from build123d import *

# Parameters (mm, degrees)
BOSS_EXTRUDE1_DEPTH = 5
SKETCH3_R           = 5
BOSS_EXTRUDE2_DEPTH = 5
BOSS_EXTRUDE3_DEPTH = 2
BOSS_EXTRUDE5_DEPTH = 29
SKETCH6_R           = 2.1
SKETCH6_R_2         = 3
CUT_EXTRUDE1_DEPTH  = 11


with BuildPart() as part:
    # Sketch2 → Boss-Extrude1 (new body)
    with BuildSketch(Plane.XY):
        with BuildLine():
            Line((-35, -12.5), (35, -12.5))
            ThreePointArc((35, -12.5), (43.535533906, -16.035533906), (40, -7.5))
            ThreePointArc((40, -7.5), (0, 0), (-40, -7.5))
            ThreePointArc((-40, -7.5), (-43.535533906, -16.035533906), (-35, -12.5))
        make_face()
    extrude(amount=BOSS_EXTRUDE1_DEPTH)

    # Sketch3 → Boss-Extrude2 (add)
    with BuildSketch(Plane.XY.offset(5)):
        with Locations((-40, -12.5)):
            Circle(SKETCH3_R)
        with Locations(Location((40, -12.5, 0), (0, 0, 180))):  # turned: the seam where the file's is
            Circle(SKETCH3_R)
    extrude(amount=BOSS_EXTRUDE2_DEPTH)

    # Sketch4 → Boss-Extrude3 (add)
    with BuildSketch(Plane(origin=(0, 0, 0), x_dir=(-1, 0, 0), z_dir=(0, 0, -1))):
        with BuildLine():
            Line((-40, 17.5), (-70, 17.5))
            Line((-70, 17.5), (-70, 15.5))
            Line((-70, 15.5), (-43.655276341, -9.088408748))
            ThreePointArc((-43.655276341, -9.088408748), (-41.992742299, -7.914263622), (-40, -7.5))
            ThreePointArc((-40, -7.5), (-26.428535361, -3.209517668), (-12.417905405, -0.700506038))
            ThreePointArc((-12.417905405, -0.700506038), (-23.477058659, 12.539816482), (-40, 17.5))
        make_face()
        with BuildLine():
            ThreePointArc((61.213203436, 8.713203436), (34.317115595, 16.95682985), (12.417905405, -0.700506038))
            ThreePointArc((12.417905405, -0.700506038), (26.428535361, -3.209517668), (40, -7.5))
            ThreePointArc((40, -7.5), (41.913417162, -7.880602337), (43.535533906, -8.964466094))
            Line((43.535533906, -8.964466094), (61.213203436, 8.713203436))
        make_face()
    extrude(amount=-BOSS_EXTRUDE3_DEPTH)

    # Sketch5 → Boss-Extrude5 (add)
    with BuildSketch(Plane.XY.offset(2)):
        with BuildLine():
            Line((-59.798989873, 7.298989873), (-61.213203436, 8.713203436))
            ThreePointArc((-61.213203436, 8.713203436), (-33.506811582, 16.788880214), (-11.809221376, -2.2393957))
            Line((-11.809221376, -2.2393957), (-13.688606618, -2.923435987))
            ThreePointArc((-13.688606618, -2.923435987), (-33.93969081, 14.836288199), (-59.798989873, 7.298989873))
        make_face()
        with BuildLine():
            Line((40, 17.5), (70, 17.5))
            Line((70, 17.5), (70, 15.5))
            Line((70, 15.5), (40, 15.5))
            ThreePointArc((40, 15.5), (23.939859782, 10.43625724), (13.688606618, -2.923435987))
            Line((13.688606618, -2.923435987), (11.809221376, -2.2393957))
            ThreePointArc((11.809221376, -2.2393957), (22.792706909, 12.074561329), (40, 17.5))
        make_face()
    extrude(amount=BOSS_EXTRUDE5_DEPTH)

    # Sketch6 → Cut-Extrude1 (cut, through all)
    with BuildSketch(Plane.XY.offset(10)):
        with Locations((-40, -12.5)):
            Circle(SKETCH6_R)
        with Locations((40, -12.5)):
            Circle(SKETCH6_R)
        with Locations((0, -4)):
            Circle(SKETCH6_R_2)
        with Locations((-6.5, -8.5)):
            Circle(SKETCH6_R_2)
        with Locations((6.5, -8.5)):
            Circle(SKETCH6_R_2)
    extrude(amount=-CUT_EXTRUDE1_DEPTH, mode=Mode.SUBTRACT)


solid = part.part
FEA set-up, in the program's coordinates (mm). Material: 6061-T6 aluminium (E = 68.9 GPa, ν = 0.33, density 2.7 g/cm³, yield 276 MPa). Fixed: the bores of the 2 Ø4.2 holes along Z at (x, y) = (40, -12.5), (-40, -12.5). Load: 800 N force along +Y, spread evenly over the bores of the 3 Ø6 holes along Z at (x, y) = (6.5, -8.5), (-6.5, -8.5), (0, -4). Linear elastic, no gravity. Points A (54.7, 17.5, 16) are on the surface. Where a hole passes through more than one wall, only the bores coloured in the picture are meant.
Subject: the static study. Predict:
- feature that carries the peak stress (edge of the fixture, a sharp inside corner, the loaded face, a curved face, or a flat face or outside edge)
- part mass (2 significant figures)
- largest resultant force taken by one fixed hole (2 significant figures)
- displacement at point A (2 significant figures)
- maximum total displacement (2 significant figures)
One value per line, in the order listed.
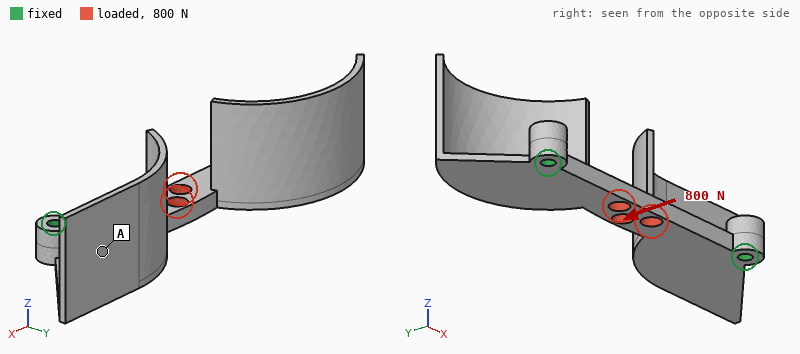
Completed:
the loaded face
41 g
670 N
61 µm
83 µm
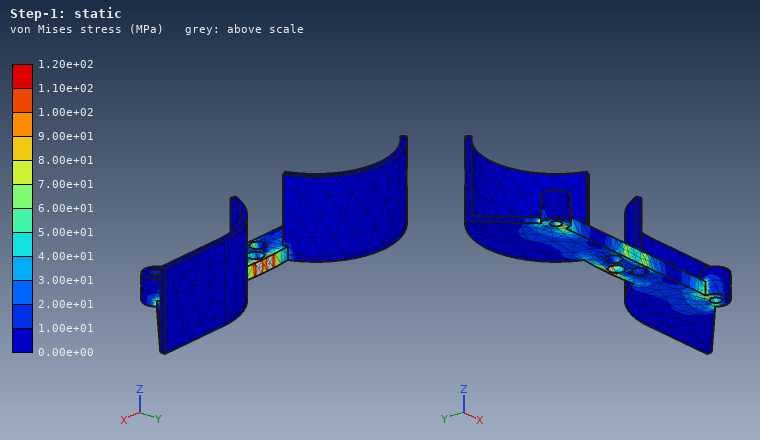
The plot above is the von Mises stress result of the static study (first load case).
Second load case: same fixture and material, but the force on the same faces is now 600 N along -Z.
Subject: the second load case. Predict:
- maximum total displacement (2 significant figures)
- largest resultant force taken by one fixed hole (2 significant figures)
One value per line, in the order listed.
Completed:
0.34 mm
310 N
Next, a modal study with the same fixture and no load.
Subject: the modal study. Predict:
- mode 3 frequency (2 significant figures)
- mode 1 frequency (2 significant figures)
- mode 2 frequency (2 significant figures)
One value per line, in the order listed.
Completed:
1200 Hz
910 Hz
1100 Hz
